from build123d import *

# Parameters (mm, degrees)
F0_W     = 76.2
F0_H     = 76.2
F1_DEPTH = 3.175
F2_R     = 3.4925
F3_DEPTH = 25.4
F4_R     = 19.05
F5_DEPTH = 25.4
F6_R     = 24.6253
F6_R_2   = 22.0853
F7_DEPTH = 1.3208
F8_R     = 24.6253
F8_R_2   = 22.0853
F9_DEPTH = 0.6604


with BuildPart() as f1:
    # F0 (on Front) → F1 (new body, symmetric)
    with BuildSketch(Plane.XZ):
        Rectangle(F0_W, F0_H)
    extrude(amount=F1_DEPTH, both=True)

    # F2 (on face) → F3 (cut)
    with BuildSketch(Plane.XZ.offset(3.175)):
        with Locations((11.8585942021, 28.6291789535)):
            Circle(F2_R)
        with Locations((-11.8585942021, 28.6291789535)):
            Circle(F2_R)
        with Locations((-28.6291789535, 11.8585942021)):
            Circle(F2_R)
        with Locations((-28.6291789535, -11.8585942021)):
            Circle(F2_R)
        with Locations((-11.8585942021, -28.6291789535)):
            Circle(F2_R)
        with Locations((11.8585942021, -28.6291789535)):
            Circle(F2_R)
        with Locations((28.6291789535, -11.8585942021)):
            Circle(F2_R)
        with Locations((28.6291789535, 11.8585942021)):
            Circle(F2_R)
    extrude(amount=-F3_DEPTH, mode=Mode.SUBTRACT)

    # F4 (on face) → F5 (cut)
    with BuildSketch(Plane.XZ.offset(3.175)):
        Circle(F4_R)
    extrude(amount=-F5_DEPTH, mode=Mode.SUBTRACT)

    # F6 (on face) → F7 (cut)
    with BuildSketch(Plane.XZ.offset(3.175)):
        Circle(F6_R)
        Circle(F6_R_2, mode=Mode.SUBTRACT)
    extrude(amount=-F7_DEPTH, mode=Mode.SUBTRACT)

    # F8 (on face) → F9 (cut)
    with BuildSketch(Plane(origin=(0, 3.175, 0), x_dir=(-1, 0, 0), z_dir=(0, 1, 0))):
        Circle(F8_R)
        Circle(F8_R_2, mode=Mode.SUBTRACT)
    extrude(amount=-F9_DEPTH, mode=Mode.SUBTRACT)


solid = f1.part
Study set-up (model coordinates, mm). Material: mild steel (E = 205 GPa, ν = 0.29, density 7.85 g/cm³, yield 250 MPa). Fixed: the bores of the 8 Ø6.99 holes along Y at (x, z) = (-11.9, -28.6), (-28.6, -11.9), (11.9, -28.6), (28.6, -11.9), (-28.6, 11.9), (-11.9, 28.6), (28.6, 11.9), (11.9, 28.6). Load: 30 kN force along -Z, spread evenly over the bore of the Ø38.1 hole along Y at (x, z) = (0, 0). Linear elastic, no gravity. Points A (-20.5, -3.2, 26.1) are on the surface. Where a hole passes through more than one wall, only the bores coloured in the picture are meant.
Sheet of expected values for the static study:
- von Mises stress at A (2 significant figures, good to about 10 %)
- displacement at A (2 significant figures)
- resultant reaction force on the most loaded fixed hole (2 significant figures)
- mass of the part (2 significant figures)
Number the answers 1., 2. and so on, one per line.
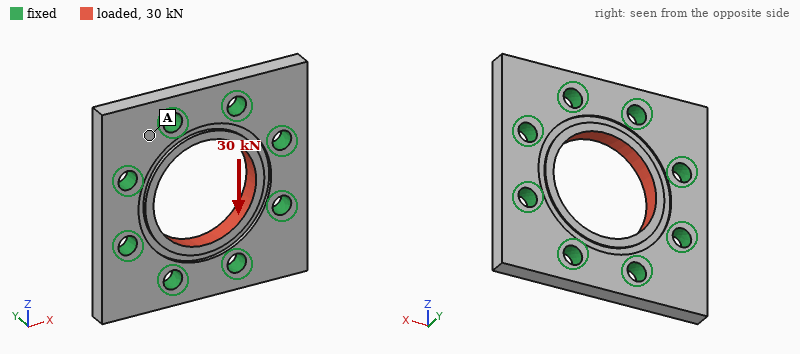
1. 13 MPa
2. 0.71 µm
3. 4.9 kN
4. 210 g
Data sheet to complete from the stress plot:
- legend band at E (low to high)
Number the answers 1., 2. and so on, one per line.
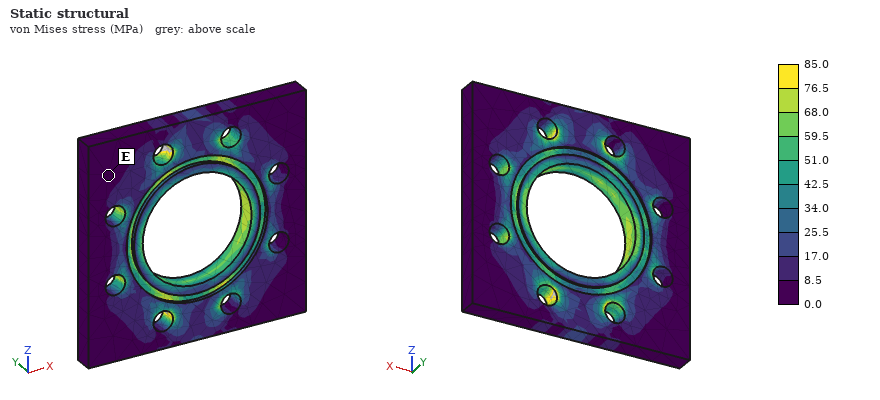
1. 0.0 to 8.5 MPa
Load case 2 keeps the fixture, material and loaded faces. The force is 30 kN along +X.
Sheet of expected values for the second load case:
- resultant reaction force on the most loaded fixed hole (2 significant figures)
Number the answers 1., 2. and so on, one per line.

1. 4.9 kN
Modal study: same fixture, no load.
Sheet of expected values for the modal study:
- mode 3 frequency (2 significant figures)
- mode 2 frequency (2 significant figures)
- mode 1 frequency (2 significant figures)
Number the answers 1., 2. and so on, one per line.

1. 15 kHz
2. 15 kHz
3. 15 kHz
